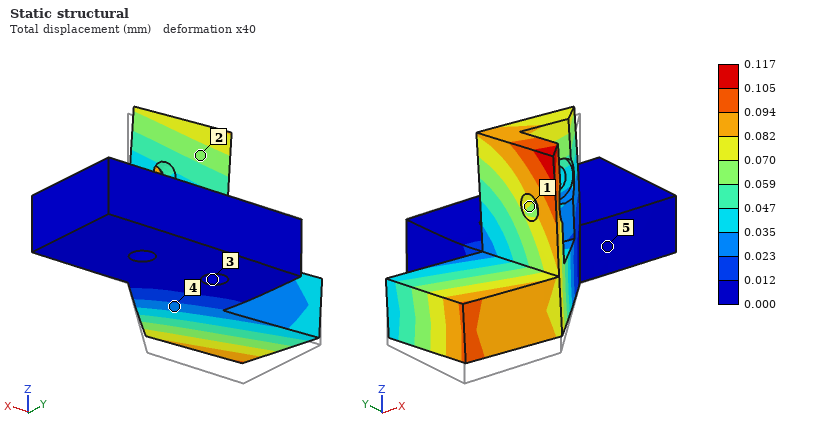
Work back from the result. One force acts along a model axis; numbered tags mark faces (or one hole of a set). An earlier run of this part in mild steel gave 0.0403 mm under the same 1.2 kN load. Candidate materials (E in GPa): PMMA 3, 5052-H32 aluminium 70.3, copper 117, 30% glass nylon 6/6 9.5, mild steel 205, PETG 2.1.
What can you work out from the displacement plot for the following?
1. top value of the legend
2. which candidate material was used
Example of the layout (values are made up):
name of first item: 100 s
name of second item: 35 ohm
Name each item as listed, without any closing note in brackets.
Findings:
top value of the legend: 0.117 mm
which candidate material was used: 5052-H32 aluminium
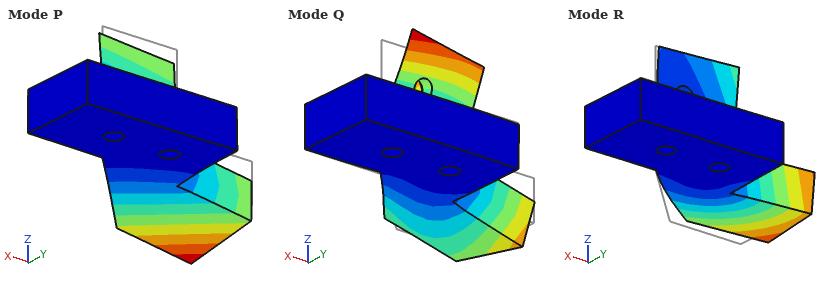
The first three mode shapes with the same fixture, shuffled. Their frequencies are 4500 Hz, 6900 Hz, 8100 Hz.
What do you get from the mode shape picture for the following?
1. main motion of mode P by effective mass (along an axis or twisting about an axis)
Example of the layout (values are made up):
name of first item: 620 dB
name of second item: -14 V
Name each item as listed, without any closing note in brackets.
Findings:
main motion of mode P by effective mass: along Z
